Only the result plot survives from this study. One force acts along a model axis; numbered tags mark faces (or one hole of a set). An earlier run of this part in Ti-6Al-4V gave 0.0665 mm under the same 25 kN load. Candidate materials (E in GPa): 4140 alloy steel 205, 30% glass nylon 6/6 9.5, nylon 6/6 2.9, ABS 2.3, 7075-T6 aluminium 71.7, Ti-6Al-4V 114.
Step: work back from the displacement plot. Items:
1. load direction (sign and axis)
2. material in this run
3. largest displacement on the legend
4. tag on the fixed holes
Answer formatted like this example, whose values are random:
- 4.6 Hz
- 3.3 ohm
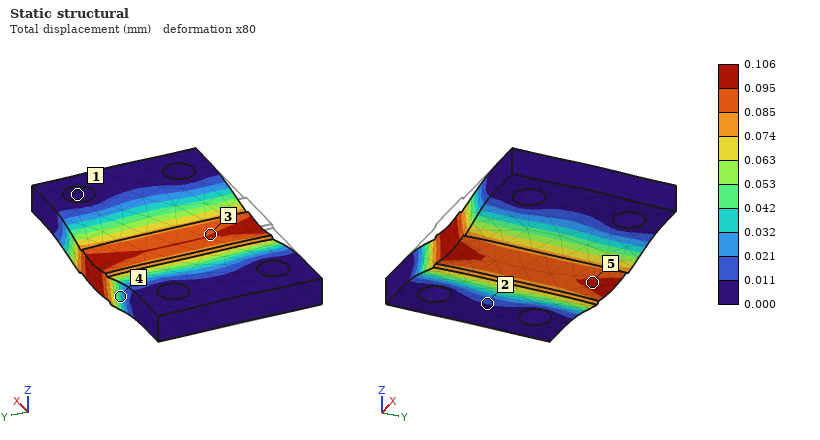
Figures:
- -Z
- 7075-T6 aluminium
- 0.106 mm
- 1
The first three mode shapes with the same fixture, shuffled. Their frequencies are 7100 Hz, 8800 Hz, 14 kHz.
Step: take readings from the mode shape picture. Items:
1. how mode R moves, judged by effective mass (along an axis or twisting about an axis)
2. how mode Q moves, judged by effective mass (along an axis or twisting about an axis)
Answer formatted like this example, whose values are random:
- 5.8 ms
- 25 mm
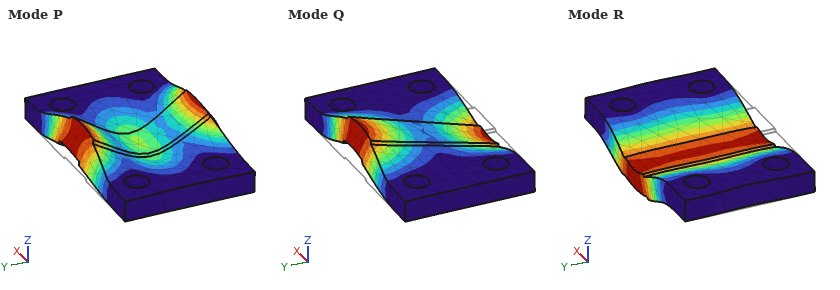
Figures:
- along Z
- twisting about X
